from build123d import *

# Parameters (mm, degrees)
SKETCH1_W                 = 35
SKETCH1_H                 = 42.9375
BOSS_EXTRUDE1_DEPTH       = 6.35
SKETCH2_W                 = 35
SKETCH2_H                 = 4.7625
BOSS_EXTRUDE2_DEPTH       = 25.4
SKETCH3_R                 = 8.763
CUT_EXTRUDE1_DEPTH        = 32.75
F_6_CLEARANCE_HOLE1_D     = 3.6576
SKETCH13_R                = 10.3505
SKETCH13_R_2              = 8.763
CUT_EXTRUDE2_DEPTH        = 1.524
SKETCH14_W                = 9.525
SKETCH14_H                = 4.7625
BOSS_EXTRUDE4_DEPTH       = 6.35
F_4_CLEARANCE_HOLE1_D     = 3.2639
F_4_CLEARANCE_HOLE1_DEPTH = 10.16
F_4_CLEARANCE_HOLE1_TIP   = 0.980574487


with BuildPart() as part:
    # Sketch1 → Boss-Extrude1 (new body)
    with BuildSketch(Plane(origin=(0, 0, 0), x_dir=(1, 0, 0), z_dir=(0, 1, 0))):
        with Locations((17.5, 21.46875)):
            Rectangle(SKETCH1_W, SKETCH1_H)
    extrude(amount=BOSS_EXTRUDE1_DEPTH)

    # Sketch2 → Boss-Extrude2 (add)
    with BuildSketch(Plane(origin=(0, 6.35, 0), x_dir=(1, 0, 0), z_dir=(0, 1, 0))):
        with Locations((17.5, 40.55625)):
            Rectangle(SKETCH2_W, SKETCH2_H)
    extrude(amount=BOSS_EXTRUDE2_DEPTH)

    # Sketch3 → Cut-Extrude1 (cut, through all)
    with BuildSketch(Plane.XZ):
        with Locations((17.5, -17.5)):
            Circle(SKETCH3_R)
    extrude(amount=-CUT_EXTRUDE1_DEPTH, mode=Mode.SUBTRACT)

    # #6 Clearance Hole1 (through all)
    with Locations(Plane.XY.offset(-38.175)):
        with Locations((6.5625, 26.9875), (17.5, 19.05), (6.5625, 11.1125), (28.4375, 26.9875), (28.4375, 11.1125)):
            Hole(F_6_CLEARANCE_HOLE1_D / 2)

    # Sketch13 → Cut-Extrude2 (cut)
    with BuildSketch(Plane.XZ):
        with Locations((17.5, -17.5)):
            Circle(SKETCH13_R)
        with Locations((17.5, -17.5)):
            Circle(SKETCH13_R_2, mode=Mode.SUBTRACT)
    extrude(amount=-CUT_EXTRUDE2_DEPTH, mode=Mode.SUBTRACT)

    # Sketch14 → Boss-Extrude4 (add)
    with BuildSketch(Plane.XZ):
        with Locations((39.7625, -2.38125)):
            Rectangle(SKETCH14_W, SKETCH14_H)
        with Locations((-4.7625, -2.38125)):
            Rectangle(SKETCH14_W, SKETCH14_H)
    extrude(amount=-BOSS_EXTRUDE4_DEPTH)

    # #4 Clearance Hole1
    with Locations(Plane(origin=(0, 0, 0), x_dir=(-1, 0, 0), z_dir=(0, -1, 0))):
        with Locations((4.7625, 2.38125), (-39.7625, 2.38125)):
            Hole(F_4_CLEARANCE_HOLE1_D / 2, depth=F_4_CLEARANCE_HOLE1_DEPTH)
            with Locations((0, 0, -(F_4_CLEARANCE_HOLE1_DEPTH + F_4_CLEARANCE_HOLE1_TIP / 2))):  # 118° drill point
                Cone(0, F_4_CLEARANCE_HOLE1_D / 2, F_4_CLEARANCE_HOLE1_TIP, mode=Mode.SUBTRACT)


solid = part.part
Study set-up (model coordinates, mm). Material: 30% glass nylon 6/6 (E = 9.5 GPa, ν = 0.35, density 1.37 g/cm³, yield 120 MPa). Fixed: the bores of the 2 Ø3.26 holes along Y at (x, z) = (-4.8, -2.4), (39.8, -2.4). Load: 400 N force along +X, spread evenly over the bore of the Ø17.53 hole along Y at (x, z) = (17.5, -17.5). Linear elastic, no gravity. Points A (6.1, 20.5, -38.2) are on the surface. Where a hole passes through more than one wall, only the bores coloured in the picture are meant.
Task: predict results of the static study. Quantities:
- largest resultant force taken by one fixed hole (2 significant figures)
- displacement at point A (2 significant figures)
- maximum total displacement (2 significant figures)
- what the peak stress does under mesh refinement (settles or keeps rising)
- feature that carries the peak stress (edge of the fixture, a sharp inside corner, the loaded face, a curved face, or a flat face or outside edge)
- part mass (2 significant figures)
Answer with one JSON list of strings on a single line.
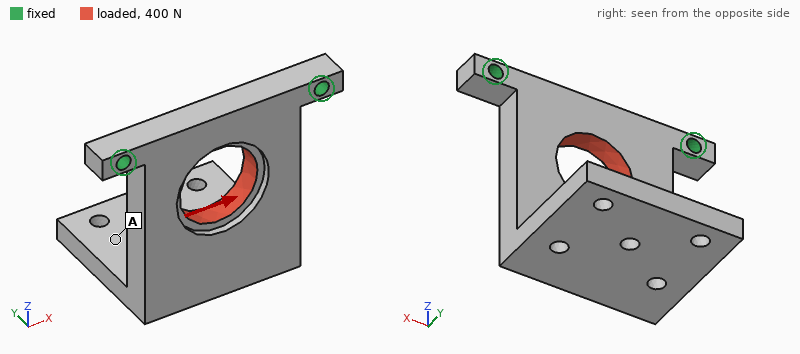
["250 N", "64 µm", "72 µm", "keeps rising", "edge of the fixture", "17 g"]
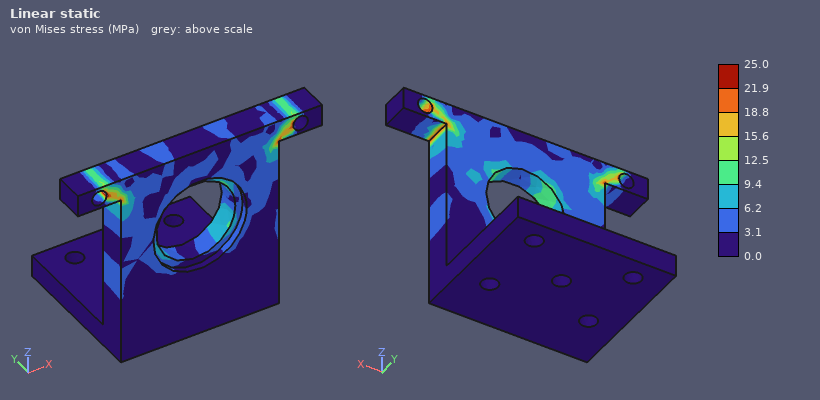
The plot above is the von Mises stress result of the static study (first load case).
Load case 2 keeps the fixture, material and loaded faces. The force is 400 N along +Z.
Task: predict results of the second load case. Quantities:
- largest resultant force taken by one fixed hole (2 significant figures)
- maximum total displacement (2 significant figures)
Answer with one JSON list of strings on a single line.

["230 N", "0.15 mm"]
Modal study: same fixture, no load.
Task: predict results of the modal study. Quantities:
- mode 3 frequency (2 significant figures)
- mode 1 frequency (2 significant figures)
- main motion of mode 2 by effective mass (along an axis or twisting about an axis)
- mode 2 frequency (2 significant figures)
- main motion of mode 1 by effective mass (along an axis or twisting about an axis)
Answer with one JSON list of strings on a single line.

["1900 Hz", "430 Hz", "along X", "1300 Hz", "along Y"]
